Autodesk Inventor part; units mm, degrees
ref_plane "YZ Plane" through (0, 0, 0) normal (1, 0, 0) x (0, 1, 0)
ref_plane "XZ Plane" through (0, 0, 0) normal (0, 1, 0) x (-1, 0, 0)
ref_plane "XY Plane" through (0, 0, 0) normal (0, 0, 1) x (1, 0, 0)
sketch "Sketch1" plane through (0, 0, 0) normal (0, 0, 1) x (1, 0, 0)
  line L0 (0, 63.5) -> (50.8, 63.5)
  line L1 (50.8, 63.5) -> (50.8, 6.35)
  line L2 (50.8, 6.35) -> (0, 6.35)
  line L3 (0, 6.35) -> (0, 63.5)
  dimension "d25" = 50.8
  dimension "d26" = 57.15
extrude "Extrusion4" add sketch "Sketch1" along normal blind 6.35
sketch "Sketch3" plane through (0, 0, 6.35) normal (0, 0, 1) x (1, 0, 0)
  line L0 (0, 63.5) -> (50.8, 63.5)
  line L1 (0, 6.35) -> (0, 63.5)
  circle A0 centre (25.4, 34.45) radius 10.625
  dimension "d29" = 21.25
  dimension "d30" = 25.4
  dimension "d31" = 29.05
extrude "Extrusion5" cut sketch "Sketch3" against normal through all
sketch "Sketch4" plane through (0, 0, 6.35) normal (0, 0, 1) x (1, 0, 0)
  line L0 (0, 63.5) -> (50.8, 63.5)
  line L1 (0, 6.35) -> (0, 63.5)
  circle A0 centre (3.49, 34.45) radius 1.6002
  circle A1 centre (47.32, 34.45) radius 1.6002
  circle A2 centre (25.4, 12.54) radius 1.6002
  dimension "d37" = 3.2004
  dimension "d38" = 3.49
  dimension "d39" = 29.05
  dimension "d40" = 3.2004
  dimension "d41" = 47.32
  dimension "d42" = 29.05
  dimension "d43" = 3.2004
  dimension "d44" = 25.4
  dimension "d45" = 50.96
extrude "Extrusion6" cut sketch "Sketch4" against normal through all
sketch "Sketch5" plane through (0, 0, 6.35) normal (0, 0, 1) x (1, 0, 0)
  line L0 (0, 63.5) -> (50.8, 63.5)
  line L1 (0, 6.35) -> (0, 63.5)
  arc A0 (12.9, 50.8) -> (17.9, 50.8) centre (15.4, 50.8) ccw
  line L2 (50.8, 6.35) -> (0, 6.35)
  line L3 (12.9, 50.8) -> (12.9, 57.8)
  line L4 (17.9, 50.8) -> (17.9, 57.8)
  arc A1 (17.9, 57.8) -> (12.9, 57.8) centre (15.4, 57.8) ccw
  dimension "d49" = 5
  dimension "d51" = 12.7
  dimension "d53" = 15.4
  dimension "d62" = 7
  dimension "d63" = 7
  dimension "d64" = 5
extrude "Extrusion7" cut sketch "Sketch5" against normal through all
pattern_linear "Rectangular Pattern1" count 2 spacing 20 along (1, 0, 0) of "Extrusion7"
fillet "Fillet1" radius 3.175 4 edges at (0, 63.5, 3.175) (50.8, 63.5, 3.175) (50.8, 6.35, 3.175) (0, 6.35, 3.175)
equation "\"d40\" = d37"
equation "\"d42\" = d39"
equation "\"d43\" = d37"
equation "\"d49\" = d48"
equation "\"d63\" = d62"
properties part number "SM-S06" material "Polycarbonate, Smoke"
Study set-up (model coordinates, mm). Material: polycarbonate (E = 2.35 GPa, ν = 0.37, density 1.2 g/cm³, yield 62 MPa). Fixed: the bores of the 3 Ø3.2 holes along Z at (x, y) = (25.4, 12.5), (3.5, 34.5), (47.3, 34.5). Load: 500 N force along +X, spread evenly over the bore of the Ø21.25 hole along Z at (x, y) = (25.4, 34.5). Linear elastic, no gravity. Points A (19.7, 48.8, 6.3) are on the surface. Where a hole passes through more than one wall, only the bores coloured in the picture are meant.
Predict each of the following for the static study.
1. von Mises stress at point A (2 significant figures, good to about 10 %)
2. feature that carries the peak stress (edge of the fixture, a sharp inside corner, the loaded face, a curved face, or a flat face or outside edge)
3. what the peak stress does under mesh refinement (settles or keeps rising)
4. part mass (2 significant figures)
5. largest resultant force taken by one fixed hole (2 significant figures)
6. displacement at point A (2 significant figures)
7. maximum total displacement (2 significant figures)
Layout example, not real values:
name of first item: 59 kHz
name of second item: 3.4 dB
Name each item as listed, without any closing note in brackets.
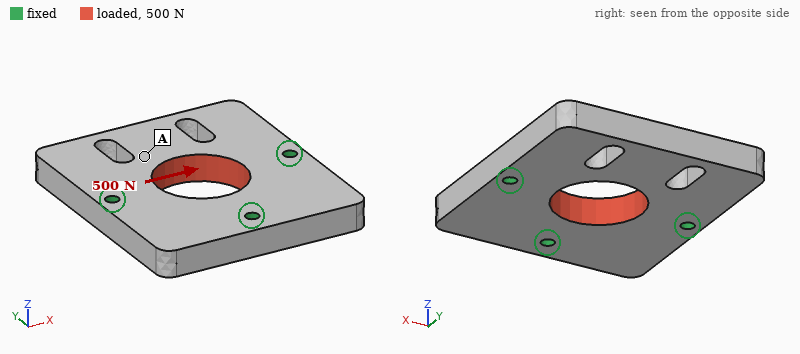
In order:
von Mises stress at point A: 0.69 MPa
feature that carries the peak stress: edge of the fixture
what the peak stress does under mesh refinement: keeps rising
part mass: 18 g
largest resultant force taken by one fixed hole: 200 N
displacement at point A: 23 µm
maximum total displacement: 28 µm
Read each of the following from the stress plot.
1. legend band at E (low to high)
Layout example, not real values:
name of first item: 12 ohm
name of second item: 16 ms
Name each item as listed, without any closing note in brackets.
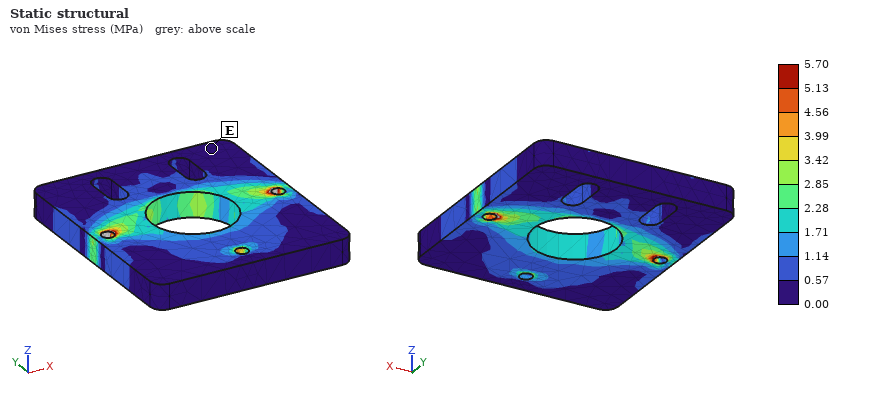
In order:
legend band at E: 0.00 to 0.57 MPa
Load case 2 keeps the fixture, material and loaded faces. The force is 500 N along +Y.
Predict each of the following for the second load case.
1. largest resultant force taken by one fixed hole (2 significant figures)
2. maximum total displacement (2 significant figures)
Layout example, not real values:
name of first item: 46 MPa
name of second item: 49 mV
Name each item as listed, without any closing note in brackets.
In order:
largest resultant force taken by one fixed hole: 170 N
maximum total displacement: 32 µm
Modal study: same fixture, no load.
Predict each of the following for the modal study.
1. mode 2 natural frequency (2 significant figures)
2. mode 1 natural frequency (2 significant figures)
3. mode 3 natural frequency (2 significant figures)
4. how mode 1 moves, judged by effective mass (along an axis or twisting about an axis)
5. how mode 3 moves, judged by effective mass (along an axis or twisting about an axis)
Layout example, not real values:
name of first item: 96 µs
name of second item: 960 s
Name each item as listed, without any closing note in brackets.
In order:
mode 2 natural frequency: 2300 Hz
mode 1 natural frequency: 1200 Hz
mode 3 natural frequency: 3400 Hz
how mode 1 moves, judged by effective mass: along Z
how mode 3 moves, judged by effective mass: twisting about Y
